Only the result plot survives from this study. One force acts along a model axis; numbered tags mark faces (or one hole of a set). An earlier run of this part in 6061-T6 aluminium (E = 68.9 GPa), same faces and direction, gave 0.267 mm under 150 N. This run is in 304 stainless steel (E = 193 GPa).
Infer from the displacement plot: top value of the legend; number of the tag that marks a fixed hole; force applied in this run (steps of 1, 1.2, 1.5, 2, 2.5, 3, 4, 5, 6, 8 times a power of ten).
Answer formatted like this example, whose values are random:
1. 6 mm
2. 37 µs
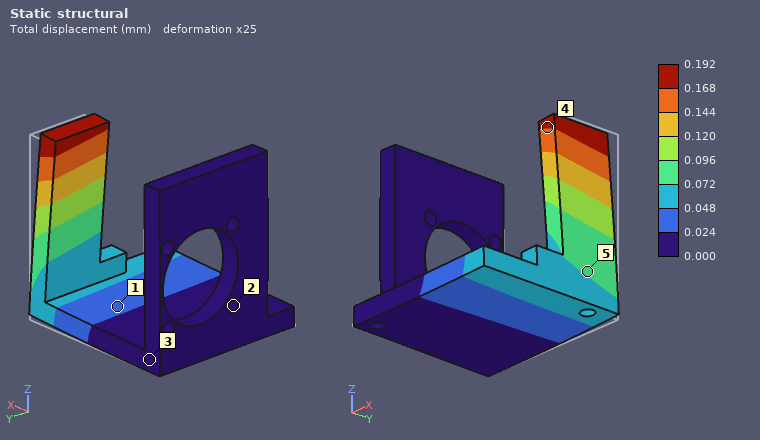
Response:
1. 0.192 mm
2. 2
3. 300 N
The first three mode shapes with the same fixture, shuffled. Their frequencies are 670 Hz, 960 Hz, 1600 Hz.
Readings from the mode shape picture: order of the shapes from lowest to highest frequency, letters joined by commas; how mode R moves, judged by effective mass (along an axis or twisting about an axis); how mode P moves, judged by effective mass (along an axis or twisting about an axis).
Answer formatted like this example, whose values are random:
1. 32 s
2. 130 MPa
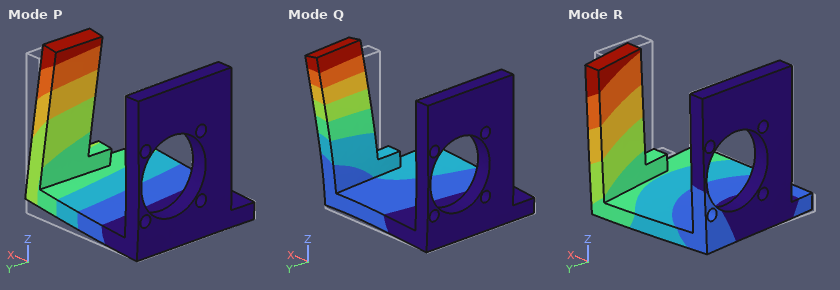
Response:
1. P, R, Q
2. along Y
3. along Z
